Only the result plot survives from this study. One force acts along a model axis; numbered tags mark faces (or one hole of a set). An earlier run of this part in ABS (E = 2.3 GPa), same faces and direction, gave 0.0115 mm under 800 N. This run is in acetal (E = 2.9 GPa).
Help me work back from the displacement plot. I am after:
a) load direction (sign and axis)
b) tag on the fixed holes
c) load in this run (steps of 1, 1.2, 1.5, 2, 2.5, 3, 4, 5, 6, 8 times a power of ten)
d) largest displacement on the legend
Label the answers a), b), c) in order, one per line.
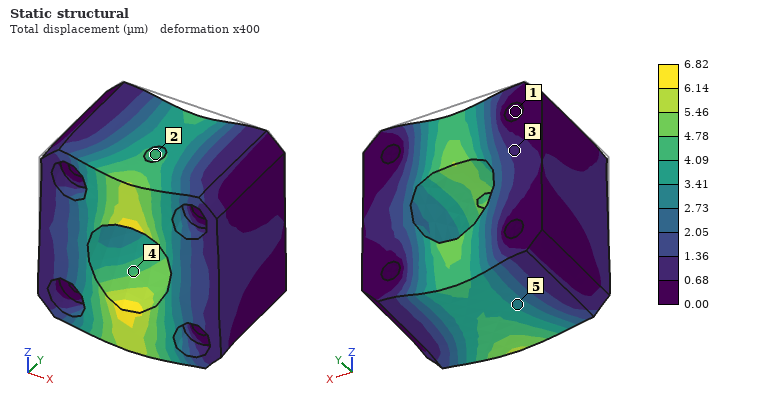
a) -Z
b) 1
c) 600 N
d) 6.82 µm
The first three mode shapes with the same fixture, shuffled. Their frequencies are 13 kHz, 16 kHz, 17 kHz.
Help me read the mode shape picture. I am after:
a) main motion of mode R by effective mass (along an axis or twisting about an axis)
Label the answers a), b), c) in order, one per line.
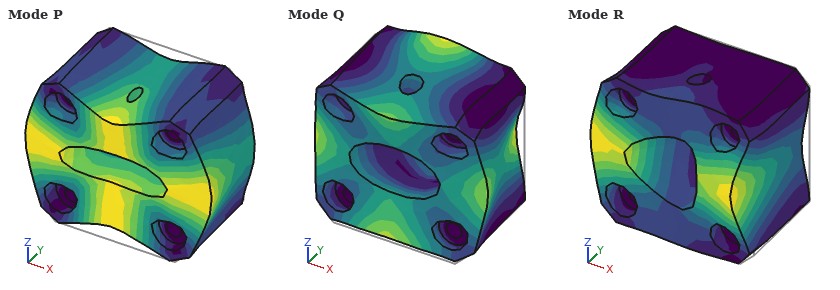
a) along X
